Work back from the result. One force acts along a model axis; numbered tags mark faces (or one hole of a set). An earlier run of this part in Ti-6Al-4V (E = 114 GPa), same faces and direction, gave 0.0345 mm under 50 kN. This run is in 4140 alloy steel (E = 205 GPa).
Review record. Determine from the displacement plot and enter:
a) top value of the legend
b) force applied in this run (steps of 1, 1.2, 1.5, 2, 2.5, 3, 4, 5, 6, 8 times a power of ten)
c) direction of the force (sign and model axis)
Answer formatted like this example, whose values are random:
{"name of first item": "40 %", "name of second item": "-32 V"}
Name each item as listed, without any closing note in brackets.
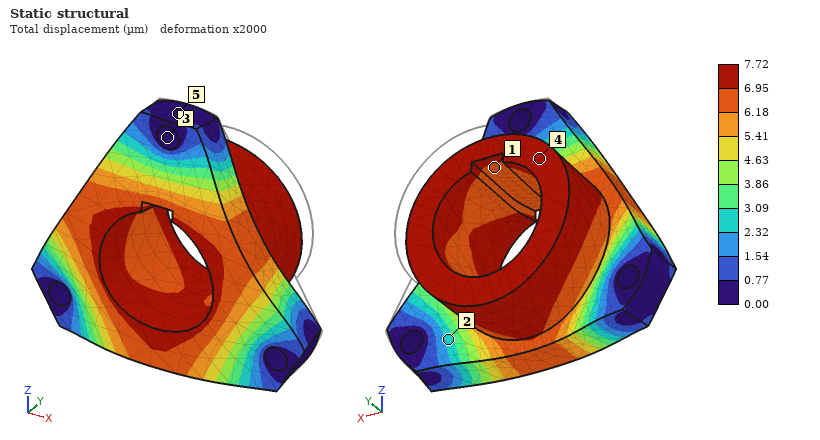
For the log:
{"top value of the legend": "7.72 µm", "force applied in this run": "20 kN", "direction of the force": "-Y"}
